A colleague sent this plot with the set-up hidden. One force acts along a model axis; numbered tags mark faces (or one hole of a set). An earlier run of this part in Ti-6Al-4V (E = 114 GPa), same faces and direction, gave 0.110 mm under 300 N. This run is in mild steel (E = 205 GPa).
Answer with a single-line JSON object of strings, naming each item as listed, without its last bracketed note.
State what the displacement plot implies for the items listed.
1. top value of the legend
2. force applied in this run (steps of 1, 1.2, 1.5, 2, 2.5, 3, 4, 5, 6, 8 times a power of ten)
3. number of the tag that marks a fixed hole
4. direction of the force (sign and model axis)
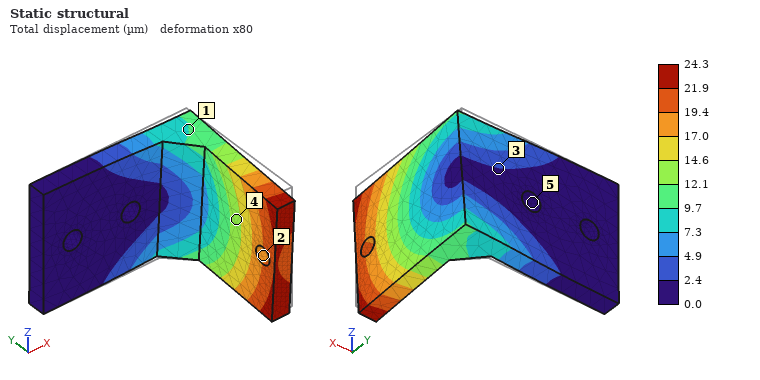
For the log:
{"top value of the legend": "24.3 µm", "force applied in this run": "120 N", "number of the tag that marks a fixed hole": "5", "direction of the force": "-Z"}
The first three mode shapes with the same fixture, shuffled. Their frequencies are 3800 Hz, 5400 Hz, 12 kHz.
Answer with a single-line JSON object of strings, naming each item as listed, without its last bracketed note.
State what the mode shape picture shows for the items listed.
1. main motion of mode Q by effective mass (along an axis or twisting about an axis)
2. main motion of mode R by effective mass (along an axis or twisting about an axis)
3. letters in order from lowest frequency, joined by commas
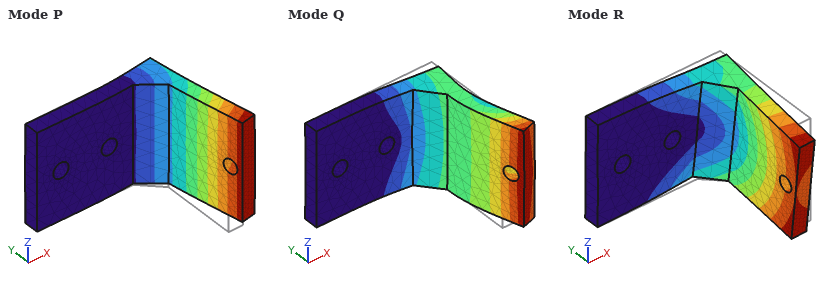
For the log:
{"main motion of mode Q by effective mass": "along Y", "main motion of mode R by effective mass": "along Z", "letters in order from lowest frequency, joined by commas": "P, R, Q"}
